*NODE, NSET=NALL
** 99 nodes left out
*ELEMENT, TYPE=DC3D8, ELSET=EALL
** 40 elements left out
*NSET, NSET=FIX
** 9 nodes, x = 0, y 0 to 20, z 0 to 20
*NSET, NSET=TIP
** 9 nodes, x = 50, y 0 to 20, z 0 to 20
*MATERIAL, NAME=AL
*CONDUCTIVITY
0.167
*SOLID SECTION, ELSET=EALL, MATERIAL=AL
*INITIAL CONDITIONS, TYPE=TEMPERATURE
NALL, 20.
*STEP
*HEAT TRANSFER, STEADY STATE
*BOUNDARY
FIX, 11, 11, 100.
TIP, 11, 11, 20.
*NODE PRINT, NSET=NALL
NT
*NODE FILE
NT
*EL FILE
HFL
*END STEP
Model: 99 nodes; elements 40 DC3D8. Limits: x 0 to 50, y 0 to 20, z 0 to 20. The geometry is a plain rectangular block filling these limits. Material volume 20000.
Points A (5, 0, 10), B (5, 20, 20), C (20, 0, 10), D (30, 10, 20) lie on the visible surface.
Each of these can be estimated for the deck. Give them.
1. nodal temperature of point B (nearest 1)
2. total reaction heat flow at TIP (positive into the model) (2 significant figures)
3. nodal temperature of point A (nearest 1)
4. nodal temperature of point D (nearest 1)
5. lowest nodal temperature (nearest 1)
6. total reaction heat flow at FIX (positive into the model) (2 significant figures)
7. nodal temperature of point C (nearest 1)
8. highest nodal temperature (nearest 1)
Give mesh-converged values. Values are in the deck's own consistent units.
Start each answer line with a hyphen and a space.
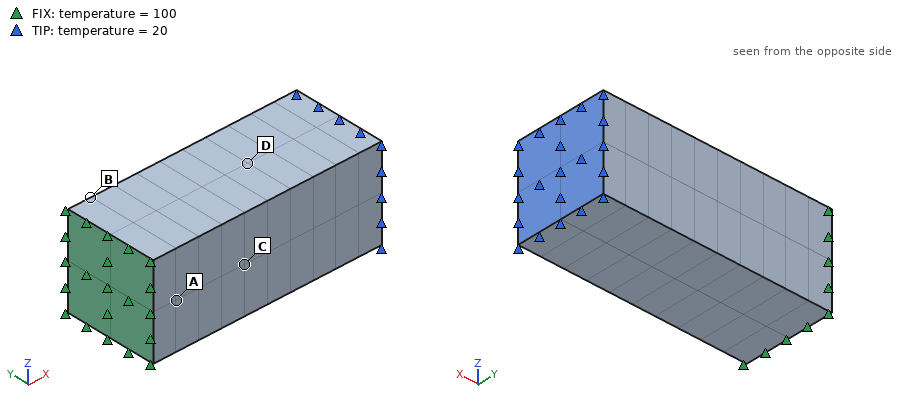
- 92
- -110
- 92
- 52
- 20
- 110
- 68
- 100
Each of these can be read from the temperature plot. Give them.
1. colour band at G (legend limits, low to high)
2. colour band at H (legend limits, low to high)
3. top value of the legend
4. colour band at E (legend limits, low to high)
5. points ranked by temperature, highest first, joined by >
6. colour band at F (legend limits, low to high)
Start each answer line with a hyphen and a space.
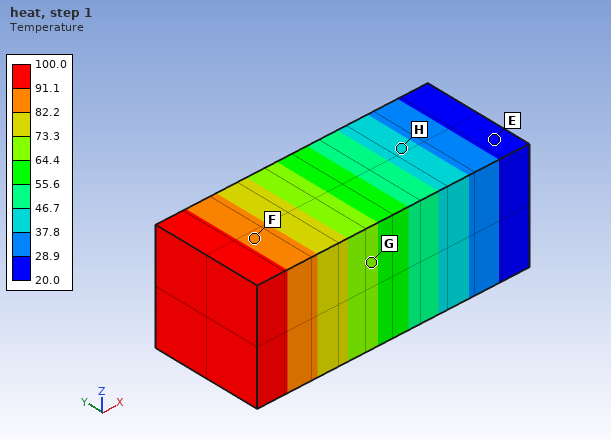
- 64.4 to 73.3
- 37.8 to 46.7
- 100.0
- 20.0 to 28.9
- F > G > H > E
- 82.2 to 91.1
